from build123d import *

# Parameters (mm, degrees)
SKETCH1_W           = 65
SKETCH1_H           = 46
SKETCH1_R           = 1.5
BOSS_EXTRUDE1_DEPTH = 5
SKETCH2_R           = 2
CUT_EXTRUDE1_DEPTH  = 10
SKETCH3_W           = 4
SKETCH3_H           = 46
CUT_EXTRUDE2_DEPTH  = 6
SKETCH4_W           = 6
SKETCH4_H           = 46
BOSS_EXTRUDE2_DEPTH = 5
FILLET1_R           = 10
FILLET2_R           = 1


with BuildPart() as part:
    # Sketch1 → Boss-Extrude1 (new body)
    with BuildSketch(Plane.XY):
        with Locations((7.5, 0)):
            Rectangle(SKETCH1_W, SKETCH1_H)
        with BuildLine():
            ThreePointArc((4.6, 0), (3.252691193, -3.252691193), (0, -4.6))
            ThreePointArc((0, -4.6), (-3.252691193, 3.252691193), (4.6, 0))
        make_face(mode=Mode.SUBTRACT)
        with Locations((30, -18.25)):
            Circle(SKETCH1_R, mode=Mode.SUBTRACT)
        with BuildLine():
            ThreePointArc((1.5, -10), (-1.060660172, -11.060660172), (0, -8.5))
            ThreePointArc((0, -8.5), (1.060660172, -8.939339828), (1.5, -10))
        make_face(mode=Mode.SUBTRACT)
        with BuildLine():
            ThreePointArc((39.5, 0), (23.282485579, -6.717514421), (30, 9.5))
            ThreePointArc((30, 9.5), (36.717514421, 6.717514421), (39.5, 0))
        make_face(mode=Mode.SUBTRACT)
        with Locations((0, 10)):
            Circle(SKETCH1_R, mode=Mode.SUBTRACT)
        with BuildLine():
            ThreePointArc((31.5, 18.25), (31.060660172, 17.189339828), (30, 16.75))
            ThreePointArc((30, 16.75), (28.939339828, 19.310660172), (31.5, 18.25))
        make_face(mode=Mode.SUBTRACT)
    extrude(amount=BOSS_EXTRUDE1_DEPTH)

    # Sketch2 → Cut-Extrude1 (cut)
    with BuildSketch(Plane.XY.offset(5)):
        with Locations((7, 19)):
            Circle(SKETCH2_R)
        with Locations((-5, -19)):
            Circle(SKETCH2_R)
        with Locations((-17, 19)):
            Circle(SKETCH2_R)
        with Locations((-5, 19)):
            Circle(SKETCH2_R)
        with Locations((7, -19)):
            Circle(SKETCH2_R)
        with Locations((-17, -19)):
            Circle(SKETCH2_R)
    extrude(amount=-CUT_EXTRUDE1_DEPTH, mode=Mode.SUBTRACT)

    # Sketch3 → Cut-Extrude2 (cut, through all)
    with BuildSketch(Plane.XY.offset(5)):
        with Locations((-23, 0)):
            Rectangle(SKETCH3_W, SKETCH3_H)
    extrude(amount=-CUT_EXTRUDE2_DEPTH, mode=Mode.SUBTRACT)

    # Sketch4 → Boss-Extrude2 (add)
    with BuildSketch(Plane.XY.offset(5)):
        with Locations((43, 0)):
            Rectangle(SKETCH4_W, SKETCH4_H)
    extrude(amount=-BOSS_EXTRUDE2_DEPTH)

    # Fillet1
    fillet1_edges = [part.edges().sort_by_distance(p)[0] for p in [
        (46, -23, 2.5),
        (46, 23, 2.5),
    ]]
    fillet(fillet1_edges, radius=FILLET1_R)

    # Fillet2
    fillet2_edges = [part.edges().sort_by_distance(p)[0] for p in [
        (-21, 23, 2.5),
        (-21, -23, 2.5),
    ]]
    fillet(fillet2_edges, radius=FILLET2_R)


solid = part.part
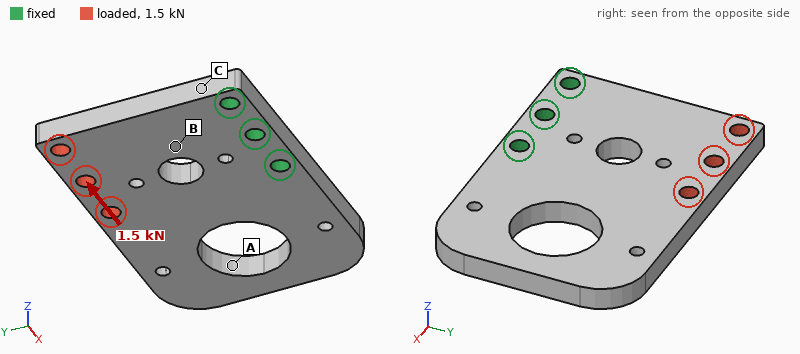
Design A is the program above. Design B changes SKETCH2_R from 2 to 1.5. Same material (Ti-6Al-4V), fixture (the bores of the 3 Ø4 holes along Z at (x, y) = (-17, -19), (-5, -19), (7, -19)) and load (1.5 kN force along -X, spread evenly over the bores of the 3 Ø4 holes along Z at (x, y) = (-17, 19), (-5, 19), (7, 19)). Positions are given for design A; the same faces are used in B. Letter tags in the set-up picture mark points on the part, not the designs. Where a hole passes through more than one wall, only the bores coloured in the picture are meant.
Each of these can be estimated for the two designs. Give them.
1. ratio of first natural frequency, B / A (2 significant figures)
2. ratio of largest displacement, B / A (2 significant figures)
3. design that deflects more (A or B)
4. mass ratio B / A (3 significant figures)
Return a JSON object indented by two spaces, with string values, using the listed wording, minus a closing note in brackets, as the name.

{
  "ratio of first natural frequency, B / A": "0.96",
  "ratio of largest displacement, B / A": "1.1",
  "design that deflects more": "B",
  "mass ratio B / A": "1.01"
}
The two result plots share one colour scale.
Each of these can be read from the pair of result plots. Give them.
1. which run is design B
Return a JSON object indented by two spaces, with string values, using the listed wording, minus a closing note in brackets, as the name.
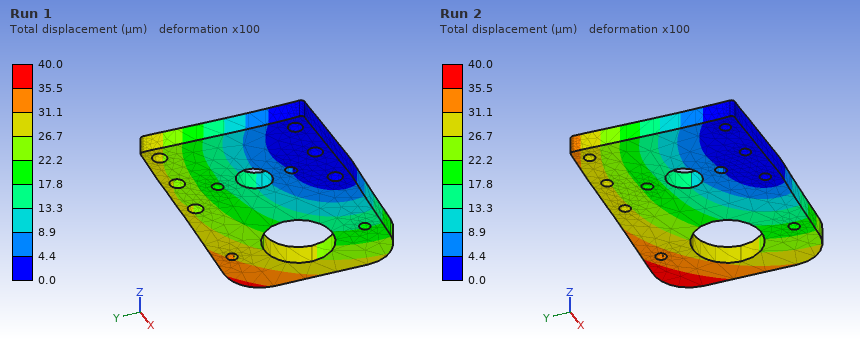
{
  "which run is design B": "Run 2"
}
